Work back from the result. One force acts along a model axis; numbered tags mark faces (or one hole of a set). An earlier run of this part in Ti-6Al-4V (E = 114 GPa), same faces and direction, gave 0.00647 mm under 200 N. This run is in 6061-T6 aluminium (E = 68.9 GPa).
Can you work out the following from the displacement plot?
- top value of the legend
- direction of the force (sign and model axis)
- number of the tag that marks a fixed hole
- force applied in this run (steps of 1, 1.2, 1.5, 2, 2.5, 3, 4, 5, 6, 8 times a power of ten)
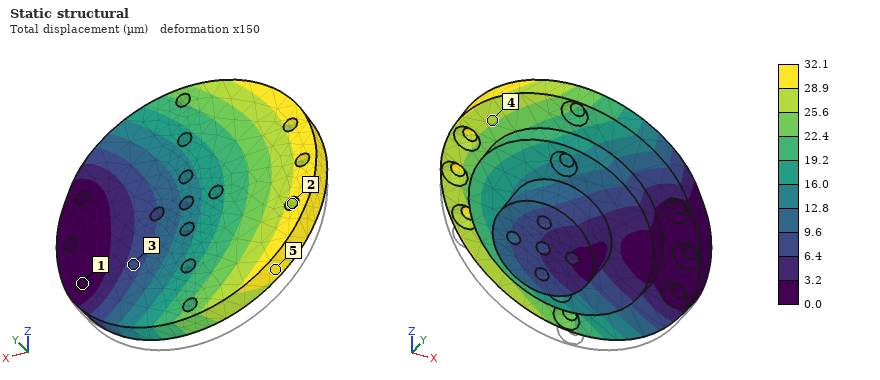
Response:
32.1 µm
+Z
1
600 N
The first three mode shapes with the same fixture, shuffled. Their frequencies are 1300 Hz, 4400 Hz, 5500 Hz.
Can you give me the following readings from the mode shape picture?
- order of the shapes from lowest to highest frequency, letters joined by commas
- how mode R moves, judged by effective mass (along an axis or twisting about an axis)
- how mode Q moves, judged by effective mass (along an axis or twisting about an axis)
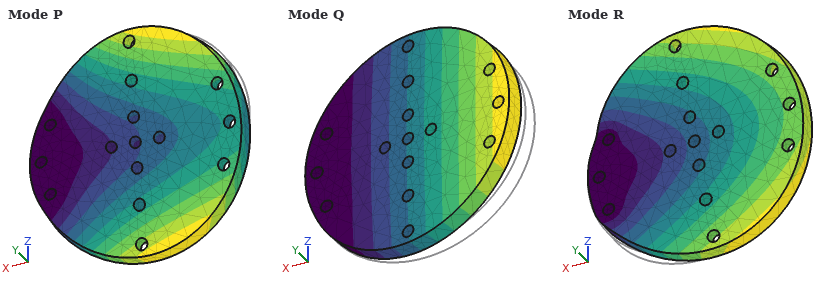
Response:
Q, P, R
along Z
along Y
